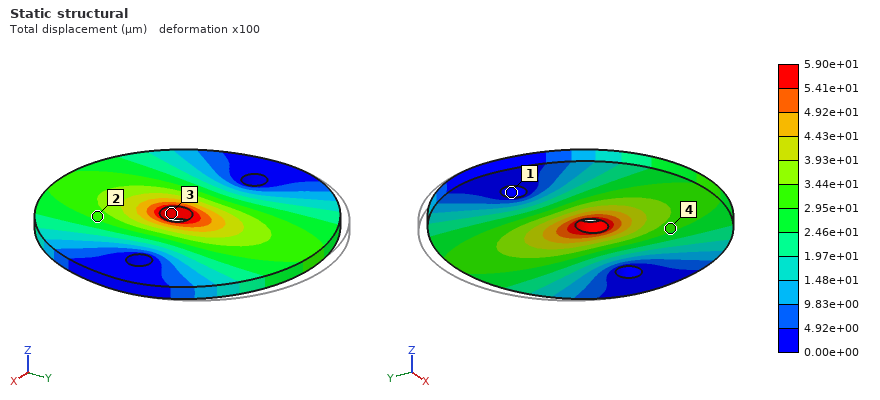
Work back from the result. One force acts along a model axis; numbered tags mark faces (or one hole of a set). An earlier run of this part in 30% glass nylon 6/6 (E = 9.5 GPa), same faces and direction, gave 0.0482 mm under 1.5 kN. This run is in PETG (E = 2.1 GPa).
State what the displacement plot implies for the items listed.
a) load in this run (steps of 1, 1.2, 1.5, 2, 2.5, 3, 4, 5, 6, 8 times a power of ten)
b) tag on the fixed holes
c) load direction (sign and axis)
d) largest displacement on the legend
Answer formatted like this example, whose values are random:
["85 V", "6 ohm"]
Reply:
["400 N", "1", "-Y", "5.90e+01 µm"]
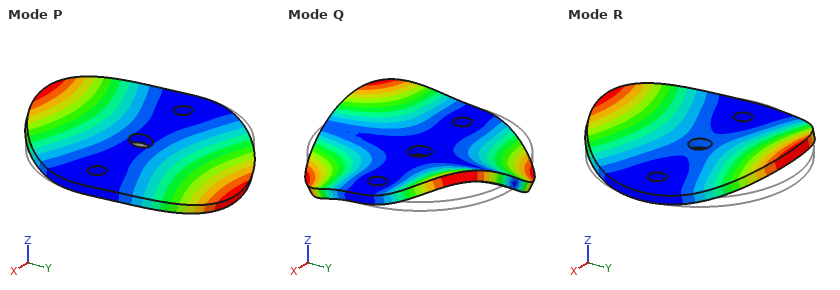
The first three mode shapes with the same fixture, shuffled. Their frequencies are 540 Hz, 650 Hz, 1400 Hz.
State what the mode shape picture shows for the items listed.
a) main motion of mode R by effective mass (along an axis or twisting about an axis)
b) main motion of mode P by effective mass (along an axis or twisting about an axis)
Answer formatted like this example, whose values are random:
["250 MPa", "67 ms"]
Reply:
["along Z", "twisting about X"]
